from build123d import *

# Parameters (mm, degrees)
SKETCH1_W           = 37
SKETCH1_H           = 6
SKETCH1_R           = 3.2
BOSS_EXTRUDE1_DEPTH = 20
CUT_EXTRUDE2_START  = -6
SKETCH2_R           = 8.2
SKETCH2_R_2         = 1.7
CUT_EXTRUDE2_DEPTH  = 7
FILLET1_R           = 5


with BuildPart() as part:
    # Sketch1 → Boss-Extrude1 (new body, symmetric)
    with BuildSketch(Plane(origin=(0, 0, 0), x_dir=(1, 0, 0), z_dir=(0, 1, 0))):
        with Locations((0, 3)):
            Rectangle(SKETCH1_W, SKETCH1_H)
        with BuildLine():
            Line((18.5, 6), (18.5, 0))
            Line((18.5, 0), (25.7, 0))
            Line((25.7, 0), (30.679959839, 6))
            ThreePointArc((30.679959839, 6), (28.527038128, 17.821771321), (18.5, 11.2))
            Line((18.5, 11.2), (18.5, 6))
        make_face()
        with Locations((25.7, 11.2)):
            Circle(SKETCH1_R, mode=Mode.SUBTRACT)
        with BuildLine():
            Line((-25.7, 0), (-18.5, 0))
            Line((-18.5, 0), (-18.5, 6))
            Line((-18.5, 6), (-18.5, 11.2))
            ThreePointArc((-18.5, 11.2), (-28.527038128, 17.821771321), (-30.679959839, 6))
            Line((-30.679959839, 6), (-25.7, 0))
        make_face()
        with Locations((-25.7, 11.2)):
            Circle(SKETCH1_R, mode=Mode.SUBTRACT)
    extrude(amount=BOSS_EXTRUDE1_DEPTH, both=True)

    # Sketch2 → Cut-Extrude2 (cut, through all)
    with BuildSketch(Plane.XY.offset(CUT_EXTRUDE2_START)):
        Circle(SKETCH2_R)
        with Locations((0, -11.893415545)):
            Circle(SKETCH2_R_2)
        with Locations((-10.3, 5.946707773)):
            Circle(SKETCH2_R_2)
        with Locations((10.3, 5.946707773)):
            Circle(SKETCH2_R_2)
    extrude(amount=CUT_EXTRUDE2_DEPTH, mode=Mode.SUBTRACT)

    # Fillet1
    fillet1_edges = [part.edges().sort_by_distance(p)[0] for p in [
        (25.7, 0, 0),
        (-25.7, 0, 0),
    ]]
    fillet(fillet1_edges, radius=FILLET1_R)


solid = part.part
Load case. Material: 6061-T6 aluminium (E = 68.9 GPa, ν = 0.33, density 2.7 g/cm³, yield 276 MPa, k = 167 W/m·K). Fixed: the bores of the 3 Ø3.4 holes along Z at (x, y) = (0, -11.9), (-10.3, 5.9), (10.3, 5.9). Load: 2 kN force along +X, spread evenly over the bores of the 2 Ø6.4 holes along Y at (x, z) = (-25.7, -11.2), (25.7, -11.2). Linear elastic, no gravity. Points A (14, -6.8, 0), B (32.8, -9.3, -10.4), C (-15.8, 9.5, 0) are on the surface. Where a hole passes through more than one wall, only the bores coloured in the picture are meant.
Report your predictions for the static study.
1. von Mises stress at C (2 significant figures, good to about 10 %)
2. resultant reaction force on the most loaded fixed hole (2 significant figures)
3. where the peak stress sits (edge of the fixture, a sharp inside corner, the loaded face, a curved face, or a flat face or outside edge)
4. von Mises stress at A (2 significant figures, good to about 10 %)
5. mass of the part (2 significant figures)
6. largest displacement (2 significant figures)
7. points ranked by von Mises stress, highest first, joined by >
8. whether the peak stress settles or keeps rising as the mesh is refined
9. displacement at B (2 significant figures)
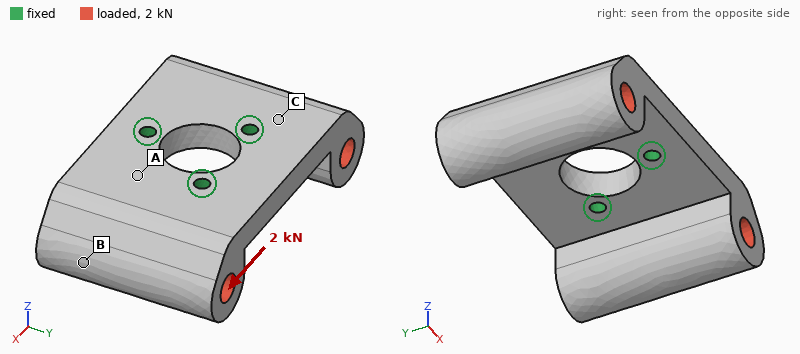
33 MPa
760 N
edge of the fixture
19 MPa
59 g
59 µm
C > A > B
keeps rising
52 µm
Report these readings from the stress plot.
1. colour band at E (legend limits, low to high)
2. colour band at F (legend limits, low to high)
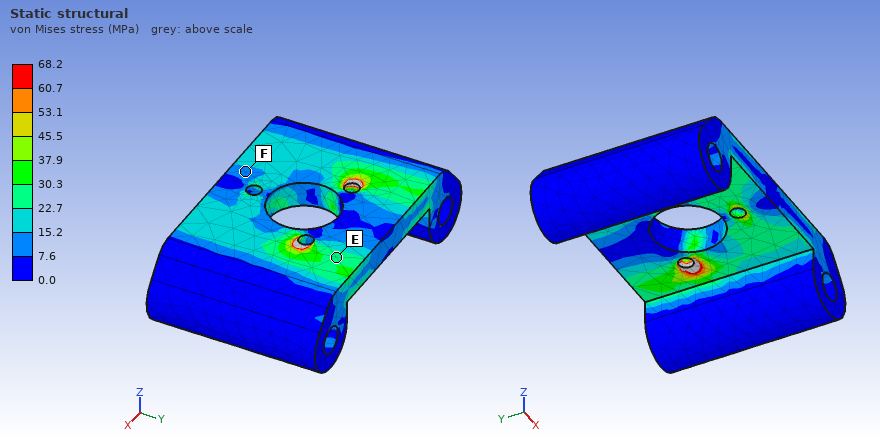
22.7 to 30.3 MPa
7.6 to 15.2 MPa
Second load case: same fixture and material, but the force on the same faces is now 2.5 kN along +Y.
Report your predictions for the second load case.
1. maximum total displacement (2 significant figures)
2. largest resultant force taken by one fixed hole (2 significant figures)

40 µm
1.1 kN
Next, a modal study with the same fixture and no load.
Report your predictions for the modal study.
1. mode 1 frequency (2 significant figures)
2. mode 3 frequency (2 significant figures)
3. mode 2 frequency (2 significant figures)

4300 Hz
7500 Hz
4300 Hz
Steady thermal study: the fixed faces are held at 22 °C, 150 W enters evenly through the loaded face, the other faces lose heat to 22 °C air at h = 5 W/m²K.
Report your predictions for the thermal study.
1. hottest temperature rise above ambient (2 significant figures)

44 K
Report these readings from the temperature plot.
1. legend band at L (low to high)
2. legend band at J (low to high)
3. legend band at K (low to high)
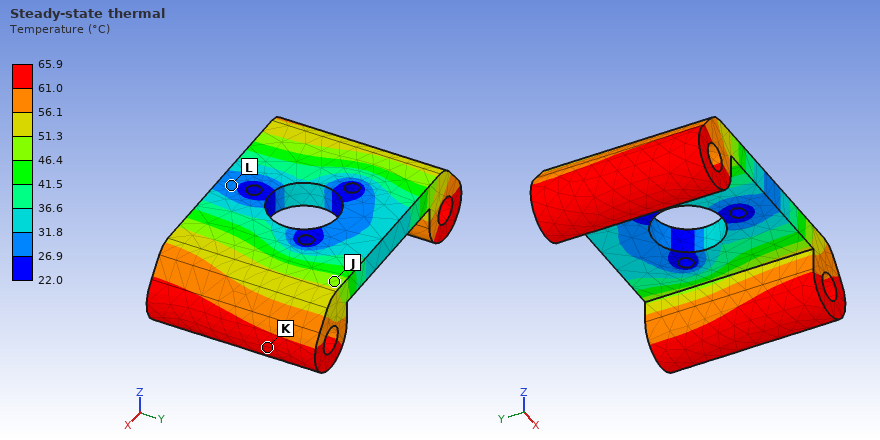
26.9 to 31.8 °C
46.4 to 51.3 °C
61.0 to 65.9 °C
